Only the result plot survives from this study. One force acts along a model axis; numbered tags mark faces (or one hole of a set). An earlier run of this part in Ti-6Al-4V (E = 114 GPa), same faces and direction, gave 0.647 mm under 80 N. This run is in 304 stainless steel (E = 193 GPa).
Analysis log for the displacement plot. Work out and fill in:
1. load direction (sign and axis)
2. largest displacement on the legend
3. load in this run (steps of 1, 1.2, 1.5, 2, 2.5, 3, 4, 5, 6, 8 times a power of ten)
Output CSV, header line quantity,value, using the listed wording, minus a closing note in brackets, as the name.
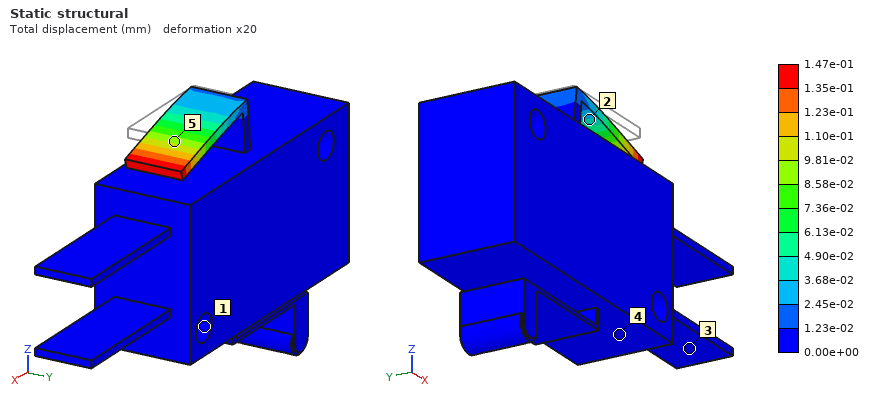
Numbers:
quantity,value
load direction,-Z
largest displacement on the legend,1.47e-01 mm
load in this run,30 N
